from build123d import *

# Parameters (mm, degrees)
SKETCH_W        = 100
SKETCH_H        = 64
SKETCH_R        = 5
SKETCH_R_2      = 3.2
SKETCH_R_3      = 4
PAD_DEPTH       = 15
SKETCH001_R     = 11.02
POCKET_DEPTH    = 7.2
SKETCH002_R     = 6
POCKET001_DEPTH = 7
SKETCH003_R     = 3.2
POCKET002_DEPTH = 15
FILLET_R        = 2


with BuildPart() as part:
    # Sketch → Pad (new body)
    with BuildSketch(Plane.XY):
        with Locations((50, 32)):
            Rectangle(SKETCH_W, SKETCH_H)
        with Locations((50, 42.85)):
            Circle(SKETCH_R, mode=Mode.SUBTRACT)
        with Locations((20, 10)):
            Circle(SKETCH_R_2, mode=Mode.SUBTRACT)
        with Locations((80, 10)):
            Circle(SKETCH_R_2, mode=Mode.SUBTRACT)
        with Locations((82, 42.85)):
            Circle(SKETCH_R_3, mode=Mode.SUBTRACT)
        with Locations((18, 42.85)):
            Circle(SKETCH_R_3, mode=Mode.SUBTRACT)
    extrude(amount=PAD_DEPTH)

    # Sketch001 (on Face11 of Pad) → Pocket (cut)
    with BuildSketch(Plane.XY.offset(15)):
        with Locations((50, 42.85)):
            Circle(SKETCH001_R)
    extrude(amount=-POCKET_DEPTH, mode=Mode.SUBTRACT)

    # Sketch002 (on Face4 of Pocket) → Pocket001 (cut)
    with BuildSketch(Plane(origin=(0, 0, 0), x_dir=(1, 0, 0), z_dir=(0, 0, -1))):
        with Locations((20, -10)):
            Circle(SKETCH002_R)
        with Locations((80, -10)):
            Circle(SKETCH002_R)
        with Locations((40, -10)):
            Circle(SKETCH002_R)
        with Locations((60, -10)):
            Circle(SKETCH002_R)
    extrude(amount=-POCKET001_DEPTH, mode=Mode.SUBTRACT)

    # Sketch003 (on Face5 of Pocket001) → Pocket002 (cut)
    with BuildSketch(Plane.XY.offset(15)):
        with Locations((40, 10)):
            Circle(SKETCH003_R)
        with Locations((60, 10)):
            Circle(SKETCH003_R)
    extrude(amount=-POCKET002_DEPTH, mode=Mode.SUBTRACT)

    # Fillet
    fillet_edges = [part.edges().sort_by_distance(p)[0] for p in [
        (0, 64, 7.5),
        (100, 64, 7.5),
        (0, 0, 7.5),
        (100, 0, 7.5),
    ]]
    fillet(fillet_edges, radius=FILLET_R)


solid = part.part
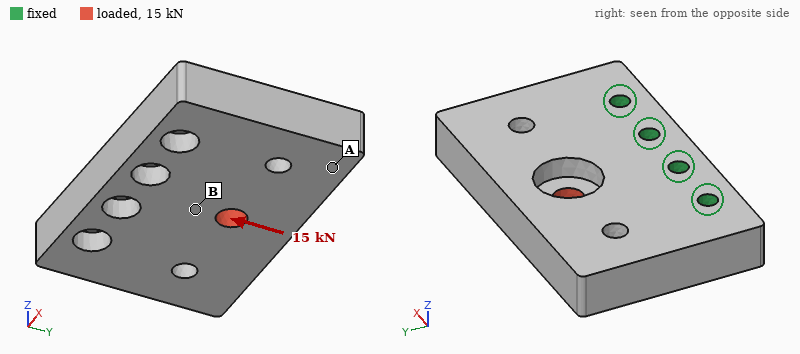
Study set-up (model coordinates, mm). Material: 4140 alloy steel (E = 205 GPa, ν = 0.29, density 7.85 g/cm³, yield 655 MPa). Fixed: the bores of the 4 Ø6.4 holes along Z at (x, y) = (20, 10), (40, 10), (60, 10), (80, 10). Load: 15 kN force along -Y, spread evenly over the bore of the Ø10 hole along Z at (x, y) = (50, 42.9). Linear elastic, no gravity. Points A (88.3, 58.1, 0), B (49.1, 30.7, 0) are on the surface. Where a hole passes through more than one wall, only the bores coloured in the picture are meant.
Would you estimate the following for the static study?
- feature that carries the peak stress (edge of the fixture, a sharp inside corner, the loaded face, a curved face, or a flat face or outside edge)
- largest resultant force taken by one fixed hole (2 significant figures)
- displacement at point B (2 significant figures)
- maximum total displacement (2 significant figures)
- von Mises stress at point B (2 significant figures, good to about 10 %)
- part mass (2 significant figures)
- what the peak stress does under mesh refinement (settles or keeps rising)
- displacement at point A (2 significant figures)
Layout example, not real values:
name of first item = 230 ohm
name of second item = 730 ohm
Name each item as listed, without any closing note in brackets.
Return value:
feature that carries the peak stress = edge of the fixture
largest resultant force taken by one fixed hole = 4.5 kN
displacement at point B = 15 µm
maximum total displacement = 37 µm
von Mises stress at point B = 53 MPa
part mass = 680 g
what the peak stress does under mesh refinement = keeps rising
displacement at point A = 28 µm
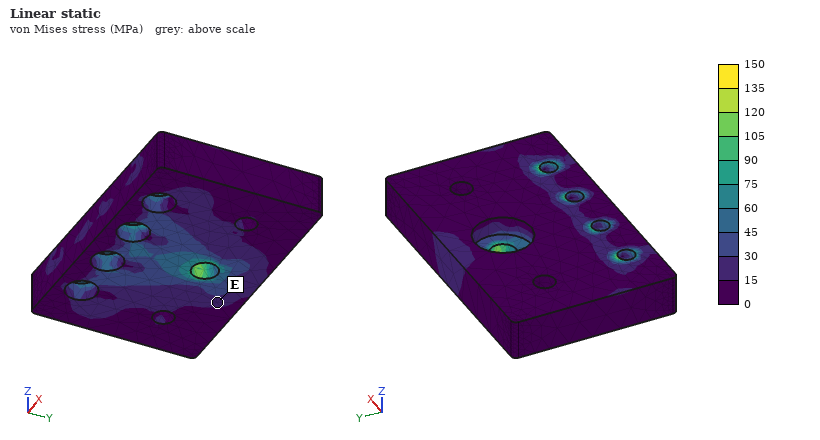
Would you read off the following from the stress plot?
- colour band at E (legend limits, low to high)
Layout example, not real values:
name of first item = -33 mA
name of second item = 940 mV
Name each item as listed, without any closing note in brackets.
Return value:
colour band at E = 15 to 30 MPa
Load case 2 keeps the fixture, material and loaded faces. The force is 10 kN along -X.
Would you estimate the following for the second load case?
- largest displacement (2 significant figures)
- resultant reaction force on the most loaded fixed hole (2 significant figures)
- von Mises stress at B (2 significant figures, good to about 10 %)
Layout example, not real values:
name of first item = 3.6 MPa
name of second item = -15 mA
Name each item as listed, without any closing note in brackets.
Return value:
largest displacement = 9.7 µm
resultant reaction force on the most loaded fixed hole = 5.4 kN
von Mises stress at B = 30 MPa
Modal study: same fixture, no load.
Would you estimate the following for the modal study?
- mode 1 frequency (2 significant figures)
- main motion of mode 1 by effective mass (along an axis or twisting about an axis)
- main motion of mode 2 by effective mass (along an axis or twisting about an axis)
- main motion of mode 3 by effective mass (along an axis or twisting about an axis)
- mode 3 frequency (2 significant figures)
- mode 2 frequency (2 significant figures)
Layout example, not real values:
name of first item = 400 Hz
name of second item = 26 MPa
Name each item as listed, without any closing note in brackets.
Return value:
mode 1 frequency = 2700 Hz
main motion of mode 1 by effective mass = along Z
main motion of mode 2 by effective mass = twisting about Y
main motion of mode 3 by effective mass = along X
mode 3 frequency = 8300 Hz
mode 2 frequency = 4400 Hz
